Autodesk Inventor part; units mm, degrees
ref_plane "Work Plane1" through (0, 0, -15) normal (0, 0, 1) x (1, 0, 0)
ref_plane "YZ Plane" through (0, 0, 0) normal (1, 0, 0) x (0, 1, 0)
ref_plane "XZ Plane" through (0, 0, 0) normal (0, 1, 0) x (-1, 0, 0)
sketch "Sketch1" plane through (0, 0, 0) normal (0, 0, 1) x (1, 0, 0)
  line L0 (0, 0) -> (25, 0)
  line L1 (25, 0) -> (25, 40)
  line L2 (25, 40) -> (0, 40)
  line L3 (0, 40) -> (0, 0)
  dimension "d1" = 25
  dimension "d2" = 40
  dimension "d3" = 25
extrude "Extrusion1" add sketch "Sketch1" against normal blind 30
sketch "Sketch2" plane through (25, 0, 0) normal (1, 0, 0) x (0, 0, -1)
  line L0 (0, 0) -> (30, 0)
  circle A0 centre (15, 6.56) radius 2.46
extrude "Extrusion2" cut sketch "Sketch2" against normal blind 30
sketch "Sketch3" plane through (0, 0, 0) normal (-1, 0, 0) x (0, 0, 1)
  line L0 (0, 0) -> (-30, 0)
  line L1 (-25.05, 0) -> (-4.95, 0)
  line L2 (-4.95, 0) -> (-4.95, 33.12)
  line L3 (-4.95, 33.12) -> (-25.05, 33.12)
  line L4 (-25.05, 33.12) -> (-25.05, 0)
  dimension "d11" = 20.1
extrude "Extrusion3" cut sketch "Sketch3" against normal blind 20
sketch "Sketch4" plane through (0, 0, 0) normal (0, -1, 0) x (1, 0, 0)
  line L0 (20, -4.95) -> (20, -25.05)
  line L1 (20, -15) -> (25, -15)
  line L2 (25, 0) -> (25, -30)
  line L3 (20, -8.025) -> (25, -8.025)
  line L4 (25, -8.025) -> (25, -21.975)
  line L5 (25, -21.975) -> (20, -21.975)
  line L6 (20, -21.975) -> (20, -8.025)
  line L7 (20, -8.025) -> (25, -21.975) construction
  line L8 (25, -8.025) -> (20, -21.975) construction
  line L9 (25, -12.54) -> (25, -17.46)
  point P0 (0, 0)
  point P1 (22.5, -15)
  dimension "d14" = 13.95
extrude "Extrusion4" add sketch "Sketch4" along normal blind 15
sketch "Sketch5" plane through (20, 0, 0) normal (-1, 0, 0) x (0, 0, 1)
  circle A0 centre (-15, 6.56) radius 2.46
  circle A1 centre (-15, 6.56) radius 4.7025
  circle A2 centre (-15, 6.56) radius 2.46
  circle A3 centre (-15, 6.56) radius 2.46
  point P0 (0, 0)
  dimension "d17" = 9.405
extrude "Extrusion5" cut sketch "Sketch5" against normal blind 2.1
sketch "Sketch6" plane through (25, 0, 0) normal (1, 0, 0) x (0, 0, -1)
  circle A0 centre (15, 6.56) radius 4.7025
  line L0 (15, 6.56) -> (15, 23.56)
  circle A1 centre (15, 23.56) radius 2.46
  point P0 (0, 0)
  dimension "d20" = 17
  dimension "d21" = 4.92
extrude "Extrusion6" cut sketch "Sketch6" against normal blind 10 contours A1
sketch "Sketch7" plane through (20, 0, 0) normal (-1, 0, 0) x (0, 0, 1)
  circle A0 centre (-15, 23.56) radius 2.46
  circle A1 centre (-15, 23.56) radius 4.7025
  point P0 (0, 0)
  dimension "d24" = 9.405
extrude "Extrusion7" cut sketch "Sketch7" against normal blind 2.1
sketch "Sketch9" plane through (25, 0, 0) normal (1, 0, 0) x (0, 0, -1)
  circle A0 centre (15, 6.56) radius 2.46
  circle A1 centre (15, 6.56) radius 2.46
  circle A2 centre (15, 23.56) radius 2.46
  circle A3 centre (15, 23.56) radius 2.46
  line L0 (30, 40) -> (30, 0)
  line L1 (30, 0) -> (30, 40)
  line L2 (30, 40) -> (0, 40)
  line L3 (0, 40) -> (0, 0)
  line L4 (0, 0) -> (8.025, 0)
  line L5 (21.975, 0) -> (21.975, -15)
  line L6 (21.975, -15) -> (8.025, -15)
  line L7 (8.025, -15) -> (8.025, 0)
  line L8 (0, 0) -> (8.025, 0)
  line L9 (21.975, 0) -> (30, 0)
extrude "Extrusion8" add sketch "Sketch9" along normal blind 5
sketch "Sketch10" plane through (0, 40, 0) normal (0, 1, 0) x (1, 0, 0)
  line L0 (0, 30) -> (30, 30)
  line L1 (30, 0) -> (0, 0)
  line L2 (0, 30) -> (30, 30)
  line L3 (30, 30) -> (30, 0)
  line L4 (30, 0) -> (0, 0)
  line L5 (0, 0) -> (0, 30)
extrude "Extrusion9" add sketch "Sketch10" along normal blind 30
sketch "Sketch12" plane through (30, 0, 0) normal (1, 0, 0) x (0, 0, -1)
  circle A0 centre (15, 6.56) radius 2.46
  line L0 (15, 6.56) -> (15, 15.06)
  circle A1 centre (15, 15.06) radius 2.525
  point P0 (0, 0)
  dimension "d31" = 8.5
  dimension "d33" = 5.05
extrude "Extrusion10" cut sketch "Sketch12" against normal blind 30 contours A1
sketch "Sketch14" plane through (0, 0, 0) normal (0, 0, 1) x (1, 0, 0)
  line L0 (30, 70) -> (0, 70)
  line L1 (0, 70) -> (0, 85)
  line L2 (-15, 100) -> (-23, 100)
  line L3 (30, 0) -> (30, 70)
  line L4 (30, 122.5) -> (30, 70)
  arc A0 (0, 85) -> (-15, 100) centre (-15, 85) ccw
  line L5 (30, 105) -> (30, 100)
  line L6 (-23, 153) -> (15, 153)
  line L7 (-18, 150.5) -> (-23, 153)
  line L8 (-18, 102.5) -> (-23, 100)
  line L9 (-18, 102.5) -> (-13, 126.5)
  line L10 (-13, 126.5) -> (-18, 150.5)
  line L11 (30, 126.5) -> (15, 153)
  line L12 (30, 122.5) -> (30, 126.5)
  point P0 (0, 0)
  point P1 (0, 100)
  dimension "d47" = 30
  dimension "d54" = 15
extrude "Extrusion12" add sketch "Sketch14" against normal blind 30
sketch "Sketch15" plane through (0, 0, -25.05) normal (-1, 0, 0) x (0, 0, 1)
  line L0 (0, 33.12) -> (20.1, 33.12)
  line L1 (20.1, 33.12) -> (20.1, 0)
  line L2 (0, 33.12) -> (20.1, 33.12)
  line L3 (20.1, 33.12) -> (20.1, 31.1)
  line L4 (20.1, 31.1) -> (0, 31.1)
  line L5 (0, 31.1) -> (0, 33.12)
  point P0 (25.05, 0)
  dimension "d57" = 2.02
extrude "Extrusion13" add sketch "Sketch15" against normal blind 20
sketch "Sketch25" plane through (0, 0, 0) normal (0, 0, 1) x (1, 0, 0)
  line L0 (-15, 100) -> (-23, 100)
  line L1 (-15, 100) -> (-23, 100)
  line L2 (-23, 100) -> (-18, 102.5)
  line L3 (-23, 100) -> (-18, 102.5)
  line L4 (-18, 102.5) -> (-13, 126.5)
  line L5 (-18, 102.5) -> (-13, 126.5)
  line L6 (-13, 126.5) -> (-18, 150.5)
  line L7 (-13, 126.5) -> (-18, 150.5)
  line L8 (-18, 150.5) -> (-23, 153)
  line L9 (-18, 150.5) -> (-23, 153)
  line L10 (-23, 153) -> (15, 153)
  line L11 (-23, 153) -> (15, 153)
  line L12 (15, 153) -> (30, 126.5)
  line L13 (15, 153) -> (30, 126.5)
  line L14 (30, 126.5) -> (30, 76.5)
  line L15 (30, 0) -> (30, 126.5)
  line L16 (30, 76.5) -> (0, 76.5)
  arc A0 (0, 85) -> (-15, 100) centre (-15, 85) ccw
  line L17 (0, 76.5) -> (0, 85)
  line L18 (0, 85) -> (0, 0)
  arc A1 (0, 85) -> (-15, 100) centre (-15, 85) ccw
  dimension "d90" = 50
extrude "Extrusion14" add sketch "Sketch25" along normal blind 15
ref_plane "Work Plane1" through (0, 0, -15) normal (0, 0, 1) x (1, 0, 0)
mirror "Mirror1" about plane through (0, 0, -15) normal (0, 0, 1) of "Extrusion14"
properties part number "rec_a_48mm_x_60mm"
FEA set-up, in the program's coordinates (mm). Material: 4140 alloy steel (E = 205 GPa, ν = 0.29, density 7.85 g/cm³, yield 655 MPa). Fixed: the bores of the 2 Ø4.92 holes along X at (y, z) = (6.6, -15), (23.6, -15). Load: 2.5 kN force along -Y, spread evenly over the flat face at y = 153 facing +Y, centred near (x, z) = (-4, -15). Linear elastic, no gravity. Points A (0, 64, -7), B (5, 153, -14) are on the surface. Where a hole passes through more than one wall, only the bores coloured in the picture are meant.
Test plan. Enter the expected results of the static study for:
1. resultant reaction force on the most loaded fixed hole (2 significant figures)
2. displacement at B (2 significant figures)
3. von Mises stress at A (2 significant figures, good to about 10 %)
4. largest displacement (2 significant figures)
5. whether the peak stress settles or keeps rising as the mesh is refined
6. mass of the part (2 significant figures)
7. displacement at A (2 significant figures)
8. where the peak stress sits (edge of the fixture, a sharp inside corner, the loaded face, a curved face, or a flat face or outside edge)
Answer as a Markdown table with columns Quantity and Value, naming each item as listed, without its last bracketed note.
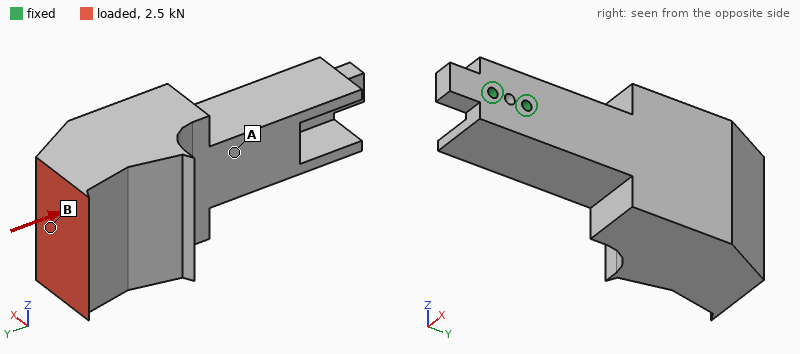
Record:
| Quantity | Value |
|---|---|
| resultant reaction force on the most loaded fixed hole | 3.4 kN |
| displacement at B | 90 µm |
| von Mises stress at A | 13 MPa |
| largest displacement | 97 µm |
| whether the peak stress settles or keeps rising as the mesh is refined | keeps rising |
| mass of the part | 1.9 kg |
| displacement at A | 29 µm |
| where the peak stress sits | edge of the fixture |
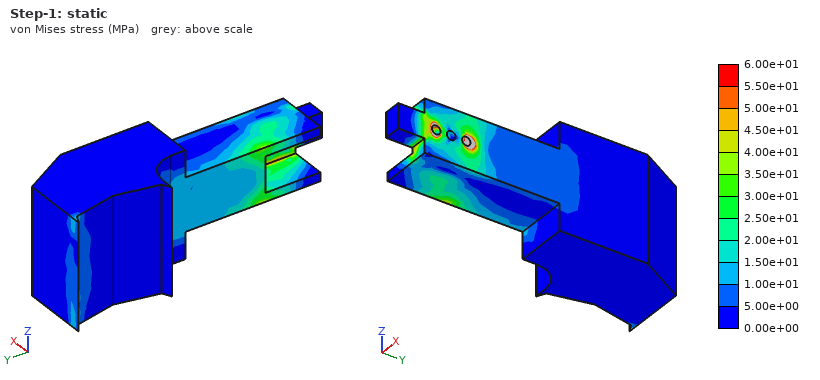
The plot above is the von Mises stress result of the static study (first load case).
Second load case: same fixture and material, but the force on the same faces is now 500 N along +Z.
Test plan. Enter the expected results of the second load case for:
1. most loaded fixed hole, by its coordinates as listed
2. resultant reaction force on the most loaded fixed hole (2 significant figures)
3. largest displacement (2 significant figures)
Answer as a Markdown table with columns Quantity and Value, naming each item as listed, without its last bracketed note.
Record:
| Quantity | Value |
|---|---|
| most loaded fixed hole, by its coordinates as listed | (23.6, -15) |
| resultant reaction force on the most loaded fixed hole | 3.3 kN |
| largest displacement | 70 µm |
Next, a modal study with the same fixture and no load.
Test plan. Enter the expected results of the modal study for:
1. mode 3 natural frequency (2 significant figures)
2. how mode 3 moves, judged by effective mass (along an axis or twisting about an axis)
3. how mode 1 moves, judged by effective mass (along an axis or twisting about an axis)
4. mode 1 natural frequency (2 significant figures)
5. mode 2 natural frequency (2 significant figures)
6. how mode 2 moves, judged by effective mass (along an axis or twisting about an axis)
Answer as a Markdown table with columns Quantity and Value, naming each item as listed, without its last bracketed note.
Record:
| Quantity | Value |
|---|---|
| mode 3 natural frequency | 1300 Hz |
| how mode 3 moves, judged by effective mass | twisting about Y |
| how mode 1 moves, judged by effective mass | along X |
| mode 1 natural frequency | 450 Hz |
| mode 2 natural frequency | 520 Hz |
| how mode 2 moves, judged by effective mass | along Z |
